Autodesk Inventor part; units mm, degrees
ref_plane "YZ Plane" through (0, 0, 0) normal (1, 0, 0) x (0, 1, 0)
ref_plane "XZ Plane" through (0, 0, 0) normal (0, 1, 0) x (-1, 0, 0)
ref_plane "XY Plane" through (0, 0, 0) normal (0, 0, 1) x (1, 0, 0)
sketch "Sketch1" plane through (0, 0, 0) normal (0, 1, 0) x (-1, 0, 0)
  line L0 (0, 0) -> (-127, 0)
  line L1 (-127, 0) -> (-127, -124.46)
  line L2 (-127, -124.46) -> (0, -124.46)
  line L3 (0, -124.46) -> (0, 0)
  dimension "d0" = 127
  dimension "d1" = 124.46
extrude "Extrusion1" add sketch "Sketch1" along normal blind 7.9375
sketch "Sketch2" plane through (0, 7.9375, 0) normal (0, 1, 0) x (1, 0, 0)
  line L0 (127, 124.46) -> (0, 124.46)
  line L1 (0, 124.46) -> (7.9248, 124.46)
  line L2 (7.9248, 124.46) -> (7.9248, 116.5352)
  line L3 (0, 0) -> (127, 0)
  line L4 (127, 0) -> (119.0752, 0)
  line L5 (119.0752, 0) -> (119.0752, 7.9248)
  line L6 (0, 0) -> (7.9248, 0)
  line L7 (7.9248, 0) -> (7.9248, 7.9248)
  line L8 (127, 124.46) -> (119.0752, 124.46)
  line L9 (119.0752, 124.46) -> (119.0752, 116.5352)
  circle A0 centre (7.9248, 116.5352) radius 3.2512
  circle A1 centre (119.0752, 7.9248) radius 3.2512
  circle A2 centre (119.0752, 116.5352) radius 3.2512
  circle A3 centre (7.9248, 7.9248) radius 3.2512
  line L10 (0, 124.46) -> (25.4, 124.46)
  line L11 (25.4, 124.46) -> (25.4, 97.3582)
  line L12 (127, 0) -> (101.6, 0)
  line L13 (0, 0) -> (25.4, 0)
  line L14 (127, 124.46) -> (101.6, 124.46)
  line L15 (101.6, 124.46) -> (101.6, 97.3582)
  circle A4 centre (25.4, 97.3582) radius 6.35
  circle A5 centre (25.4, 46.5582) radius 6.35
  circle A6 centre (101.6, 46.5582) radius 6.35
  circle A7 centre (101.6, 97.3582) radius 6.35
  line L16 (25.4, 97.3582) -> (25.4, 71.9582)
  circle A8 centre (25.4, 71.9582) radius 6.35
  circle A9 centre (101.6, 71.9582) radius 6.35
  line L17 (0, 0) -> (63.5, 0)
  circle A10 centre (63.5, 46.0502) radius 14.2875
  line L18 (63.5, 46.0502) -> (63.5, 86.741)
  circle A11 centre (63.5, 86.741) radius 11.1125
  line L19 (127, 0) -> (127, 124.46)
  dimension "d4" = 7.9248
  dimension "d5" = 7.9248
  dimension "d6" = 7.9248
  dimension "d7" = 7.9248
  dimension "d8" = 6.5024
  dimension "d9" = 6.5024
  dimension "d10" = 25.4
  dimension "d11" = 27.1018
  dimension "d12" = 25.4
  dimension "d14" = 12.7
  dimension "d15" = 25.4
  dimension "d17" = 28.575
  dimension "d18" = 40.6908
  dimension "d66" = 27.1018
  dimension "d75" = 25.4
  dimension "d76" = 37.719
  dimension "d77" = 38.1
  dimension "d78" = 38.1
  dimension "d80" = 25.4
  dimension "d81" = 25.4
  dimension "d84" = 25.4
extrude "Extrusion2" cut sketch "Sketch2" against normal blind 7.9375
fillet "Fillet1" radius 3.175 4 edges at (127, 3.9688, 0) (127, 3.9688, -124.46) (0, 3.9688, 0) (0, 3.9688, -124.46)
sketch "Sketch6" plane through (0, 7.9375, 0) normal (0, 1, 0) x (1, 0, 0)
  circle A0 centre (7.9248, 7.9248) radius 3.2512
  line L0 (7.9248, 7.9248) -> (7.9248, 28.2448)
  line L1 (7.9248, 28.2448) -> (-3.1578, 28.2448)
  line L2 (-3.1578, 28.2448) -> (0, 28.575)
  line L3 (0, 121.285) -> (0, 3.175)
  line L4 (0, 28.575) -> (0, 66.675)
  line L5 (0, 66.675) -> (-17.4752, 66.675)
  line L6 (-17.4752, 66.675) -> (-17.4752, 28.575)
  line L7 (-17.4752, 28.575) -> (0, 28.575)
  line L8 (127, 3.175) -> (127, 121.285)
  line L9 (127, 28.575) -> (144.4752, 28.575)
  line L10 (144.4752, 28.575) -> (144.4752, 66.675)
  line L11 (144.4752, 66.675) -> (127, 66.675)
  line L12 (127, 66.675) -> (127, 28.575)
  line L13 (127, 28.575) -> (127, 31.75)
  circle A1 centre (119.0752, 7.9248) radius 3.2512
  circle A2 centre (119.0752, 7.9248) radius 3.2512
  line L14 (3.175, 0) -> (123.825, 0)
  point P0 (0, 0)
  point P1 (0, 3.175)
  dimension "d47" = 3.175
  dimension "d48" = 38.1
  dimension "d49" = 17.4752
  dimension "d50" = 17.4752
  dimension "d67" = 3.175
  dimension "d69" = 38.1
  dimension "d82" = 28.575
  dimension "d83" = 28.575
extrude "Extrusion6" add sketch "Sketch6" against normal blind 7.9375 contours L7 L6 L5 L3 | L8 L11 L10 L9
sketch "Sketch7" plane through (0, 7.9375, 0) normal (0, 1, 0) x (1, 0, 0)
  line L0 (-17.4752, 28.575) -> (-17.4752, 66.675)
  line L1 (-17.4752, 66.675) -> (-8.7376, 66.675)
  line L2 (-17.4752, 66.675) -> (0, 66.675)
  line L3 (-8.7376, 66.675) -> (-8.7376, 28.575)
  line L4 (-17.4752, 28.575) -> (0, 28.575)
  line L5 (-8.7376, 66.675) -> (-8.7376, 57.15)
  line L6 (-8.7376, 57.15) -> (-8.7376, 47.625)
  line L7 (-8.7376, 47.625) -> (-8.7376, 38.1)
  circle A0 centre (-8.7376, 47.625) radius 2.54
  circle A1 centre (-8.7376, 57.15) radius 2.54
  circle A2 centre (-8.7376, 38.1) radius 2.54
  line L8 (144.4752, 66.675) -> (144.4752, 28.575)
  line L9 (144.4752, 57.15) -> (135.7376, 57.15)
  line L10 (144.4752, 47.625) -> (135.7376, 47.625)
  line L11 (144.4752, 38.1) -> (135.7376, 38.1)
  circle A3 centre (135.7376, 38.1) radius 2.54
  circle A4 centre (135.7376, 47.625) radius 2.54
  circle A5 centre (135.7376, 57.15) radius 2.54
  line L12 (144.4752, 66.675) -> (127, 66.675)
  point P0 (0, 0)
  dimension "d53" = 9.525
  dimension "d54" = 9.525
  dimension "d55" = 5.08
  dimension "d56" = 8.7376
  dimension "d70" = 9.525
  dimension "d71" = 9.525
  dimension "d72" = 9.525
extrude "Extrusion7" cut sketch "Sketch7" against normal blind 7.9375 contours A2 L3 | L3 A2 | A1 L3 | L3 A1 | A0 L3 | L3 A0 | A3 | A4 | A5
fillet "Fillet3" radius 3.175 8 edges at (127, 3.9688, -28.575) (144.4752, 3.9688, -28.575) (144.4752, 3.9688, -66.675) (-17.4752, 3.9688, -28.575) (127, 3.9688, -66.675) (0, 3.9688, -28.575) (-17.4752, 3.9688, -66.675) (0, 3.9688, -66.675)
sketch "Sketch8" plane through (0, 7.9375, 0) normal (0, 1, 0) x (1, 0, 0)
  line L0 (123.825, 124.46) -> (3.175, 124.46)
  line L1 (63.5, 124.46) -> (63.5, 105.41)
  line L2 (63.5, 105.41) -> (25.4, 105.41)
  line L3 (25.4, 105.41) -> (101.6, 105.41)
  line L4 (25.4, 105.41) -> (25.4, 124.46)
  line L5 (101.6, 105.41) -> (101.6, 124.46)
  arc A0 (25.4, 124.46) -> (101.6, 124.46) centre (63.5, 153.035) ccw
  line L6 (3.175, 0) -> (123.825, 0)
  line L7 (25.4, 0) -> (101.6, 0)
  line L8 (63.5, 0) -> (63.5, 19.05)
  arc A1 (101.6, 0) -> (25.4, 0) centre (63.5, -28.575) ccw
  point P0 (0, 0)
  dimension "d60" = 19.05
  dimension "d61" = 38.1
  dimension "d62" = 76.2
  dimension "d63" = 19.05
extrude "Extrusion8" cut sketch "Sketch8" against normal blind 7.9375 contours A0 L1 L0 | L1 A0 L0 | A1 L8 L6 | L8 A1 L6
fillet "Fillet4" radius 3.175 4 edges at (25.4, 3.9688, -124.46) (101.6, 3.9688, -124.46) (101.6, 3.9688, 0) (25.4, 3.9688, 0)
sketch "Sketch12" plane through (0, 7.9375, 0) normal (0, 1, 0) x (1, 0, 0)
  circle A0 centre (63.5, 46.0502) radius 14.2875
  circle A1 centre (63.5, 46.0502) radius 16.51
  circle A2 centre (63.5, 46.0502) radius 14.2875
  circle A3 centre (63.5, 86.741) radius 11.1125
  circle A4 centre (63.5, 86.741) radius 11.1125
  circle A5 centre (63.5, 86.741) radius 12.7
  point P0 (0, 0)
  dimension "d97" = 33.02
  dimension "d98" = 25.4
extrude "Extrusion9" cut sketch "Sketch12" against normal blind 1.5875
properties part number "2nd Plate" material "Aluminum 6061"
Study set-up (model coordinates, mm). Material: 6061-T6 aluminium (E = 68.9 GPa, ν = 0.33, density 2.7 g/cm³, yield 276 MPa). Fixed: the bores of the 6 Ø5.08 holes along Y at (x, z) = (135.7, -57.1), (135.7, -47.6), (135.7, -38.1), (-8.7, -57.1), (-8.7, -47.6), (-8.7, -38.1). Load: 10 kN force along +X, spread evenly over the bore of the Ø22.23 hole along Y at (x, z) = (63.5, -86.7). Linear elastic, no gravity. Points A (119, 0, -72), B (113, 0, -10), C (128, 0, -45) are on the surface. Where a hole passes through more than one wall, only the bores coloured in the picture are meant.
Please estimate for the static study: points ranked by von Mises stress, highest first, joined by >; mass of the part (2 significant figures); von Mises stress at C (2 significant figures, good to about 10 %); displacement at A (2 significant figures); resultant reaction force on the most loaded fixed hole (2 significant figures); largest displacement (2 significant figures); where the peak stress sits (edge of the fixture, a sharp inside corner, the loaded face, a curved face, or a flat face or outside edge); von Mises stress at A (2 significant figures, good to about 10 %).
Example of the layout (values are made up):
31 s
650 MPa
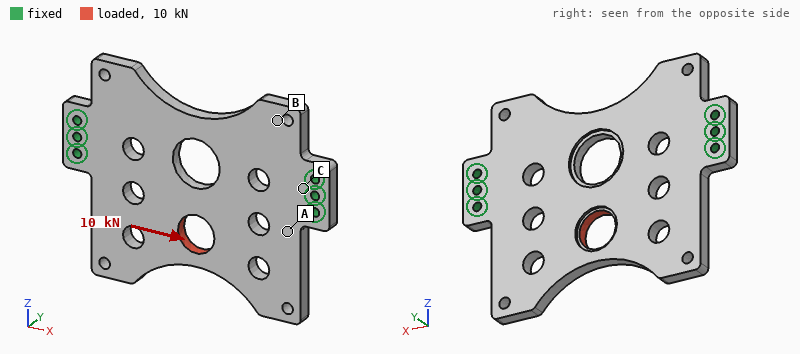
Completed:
A > C > B
280 g
12 MPa
13 µm
3.0 kN
45 µm
a curved face
28 MPa
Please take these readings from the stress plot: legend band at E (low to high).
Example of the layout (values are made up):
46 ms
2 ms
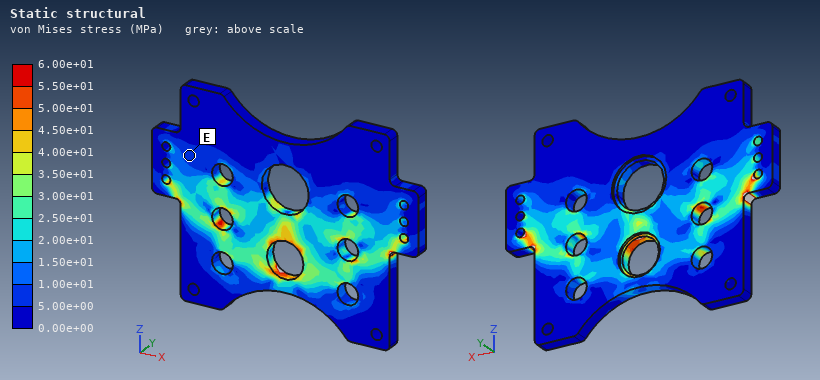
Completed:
5.00e+00 to 1.00e+01 MPa
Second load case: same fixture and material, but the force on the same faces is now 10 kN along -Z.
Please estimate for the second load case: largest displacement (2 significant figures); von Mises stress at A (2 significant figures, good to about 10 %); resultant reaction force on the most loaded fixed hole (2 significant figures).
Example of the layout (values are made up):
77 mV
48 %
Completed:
96 µm
29 MPa
3.1 kN
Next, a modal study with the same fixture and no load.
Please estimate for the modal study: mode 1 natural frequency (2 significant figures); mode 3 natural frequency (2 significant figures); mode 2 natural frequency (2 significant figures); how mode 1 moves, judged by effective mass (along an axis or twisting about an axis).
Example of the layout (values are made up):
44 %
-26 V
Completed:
960 Hz
1700 Hz
1700 Hz
along Y
